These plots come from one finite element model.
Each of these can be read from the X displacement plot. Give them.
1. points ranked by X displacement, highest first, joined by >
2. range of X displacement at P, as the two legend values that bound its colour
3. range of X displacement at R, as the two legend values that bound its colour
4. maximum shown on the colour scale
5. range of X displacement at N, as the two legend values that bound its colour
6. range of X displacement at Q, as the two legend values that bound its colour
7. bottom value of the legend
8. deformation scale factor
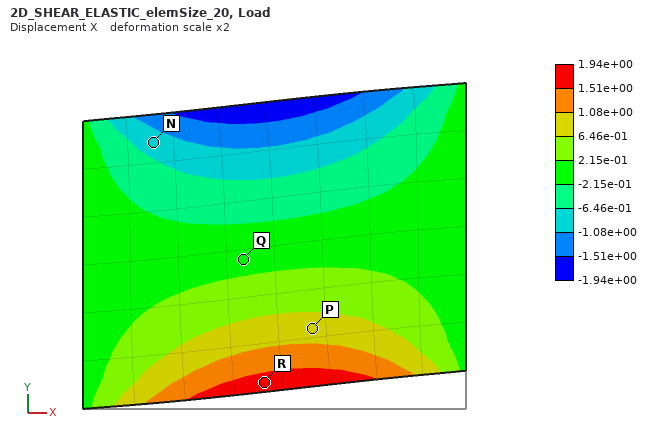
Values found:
R > P > Q > N
6.46e-01 to 1.08e+00
1.51e+00 to 1.94e+00
1.94e+00
-1.08e+00 to -6.46e-01
-2.15e-01 to 2.15e-01
-1.94e+00
2
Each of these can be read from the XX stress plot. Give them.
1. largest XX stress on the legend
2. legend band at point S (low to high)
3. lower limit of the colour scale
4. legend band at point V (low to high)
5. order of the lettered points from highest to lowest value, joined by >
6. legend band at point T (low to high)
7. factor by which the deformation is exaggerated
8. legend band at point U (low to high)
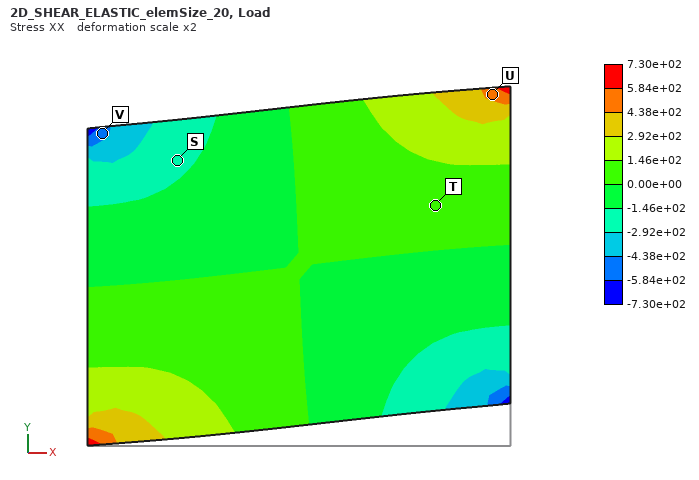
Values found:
7.30e+02
-2.92e+02 to -1.46e+02
-7.30e+02
-5.84e+02 to -4.38e+02
U > T > S > V
0.00e+00 to 1.46e+02
2
4.38e+02 to 5.84e+02
